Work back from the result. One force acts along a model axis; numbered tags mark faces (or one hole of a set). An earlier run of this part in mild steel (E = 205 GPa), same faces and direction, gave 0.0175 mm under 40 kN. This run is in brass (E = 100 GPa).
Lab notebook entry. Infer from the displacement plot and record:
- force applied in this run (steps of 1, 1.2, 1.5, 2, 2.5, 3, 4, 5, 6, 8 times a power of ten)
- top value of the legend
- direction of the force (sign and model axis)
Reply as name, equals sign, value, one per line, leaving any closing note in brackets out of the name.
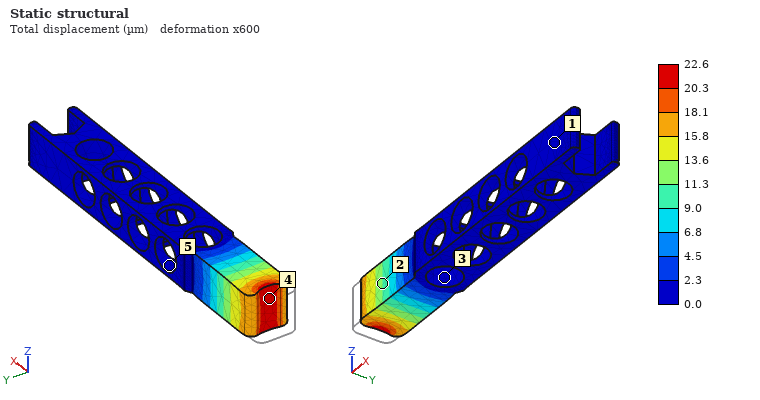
force applied in this run = 25 kN
top value of the legend = 22.6 µm
direction of the force = +X
